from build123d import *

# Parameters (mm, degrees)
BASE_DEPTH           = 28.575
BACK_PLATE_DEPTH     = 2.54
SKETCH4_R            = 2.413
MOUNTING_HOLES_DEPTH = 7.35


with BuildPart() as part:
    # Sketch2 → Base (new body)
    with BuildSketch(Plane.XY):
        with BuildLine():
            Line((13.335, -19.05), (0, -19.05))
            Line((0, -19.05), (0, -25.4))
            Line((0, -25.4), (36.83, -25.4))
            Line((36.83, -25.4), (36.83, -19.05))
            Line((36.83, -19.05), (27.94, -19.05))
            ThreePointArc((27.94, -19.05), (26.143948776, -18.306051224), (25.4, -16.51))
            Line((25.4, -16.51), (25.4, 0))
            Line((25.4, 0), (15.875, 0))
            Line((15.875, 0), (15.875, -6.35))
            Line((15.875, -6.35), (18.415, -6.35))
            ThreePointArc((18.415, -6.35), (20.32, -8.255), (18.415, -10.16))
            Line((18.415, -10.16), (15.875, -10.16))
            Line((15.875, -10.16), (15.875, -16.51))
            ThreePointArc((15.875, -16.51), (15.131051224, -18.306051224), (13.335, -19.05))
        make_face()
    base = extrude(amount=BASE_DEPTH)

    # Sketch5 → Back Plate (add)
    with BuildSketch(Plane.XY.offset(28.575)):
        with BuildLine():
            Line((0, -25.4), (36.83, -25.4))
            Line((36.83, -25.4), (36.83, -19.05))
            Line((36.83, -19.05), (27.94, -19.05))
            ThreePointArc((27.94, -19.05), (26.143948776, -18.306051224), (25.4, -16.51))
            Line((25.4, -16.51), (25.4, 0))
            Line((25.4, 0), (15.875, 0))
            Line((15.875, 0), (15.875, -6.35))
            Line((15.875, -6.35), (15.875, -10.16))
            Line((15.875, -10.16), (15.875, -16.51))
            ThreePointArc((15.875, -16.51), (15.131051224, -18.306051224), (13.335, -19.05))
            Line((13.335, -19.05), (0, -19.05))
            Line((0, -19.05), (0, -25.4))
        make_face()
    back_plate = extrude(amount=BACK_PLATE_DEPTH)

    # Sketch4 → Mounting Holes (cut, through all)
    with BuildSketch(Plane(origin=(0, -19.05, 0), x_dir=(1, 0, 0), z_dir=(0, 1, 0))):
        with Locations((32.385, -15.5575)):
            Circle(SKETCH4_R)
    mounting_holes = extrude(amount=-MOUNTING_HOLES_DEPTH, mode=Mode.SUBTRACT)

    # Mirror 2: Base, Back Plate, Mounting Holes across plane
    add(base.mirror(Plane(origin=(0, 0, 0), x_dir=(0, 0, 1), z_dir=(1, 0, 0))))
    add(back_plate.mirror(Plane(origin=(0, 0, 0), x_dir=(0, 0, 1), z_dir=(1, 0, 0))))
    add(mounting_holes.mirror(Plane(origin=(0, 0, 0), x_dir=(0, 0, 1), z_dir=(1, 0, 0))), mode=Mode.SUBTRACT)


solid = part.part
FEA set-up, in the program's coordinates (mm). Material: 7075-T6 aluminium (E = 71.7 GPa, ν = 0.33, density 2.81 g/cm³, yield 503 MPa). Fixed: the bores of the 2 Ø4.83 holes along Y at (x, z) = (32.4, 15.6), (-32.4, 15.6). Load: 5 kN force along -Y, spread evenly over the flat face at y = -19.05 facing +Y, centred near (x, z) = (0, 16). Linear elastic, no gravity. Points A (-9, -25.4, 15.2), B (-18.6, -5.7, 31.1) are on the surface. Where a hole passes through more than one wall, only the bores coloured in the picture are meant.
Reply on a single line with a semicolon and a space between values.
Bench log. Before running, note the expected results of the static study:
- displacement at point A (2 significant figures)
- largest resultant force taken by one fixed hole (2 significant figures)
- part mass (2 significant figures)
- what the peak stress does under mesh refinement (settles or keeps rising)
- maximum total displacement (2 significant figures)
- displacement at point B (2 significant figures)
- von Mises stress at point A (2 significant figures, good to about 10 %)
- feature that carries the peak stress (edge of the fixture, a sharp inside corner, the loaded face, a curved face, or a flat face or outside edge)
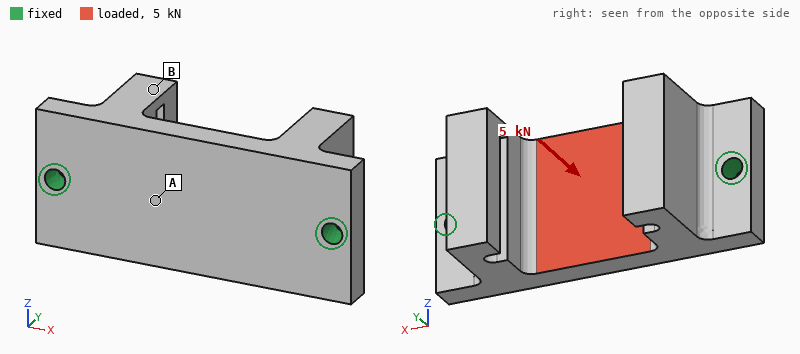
0.14 mm; 2.5 kN; 70 g; keeps rising; 0.18 mm; 0.13 mm; 90 MPa; edge of the fixture
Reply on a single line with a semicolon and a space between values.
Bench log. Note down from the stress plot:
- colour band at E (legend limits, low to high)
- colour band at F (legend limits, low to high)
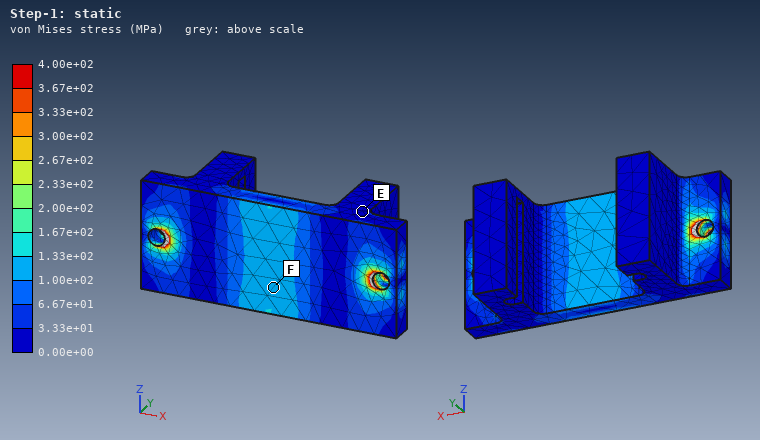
0.00e+00 to 3.33e+01 MPa; 1.00e+02 to 1.33e+02 MPa
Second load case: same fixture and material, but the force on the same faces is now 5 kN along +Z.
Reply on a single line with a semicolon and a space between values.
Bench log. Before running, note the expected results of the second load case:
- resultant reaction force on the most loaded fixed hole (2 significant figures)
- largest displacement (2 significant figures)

2.5 kN; 47 µm
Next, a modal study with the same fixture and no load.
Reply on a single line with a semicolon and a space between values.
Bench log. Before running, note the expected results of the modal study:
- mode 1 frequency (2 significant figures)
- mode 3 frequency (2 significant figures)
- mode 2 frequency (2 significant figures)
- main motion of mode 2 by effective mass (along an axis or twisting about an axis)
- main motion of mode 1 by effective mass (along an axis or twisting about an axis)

4700 Hz; 7800 Hz; 5400 Hz; along Z; along Y
